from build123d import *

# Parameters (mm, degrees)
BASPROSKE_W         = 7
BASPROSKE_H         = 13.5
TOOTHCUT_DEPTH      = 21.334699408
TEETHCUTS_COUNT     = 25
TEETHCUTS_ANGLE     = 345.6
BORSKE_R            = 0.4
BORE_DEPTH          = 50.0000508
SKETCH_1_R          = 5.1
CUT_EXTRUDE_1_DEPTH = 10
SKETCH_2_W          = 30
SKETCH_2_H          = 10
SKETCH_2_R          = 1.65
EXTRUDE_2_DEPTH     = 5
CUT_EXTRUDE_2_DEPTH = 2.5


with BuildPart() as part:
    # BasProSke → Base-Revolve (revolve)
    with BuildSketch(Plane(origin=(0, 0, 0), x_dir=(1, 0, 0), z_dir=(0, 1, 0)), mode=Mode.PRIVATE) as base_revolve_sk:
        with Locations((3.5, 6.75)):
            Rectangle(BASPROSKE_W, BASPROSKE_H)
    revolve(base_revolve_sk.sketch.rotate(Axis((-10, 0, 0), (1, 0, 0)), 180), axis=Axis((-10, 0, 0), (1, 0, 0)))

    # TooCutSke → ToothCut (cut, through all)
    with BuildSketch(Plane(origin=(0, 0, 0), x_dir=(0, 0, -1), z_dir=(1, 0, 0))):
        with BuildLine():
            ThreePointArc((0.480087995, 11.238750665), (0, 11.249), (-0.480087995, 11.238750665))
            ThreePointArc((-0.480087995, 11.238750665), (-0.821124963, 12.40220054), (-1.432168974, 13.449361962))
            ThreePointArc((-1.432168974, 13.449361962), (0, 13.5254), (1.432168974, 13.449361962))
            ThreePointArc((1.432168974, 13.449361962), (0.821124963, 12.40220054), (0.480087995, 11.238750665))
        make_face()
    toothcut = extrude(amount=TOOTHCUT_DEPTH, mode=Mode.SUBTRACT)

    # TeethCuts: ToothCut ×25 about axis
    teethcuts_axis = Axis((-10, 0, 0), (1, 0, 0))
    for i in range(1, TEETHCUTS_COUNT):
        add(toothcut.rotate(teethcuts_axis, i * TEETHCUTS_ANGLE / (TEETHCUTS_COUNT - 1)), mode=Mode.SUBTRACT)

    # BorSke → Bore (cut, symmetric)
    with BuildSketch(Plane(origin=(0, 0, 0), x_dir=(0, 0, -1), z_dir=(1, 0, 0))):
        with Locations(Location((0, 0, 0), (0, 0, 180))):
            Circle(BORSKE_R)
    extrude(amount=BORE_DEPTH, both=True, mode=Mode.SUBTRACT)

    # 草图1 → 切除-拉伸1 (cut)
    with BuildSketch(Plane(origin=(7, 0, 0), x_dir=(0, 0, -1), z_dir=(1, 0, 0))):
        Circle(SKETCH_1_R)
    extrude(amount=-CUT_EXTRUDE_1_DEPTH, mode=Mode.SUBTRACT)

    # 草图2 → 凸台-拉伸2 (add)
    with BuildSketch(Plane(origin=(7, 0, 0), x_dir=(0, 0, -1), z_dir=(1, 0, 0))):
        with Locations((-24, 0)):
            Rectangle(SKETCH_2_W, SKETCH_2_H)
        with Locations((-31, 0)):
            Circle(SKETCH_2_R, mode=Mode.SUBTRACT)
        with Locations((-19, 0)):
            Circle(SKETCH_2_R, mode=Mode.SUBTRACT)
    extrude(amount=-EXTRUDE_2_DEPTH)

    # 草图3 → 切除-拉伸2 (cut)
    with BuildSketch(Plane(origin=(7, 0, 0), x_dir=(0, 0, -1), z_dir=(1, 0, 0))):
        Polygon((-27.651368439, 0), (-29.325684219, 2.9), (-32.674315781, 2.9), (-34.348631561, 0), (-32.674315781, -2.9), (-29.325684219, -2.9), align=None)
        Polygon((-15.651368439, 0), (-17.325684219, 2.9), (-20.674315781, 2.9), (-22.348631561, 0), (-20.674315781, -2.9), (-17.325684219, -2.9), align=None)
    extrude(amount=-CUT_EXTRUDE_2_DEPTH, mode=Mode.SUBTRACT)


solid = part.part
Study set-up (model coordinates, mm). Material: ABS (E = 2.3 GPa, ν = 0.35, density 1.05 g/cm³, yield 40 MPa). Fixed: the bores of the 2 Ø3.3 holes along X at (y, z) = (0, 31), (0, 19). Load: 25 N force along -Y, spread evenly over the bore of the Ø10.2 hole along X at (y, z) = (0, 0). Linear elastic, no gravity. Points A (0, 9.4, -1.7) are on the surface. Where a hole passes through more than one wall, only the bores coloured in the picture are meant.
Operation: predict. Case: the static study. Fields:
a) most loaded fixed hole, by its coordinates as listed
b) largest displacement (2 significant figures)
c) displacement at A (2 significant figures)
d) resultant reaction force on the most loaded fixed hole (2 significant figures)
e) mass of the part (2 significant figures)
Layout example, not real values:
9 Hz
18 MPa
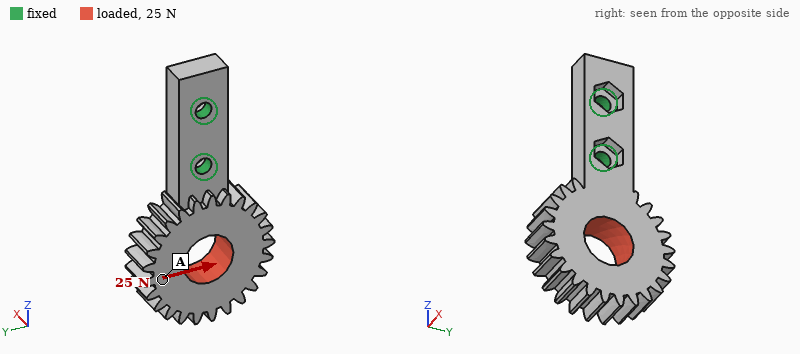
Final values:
(0, 19)
0.20 mm
0.14 mm
48 N
4.1 g
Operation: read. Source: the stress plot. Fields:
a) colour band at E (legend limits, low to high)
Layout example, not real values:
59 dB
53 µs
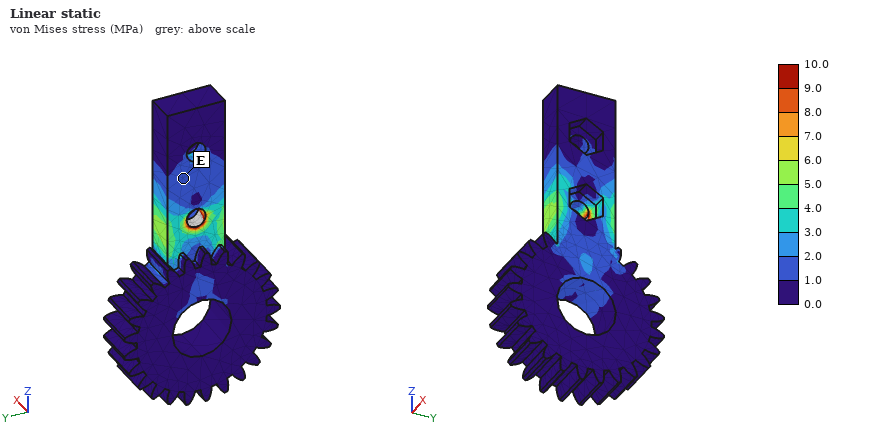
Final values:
1.0 to 2.0 MPa
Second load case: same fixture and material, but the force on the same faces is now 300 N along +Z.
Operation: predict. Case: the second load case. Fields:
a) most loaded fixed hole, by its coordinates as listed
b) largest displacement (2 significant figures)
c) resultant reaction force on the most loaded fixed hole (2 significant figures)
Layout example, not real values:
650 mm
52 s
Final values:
(0, 19)
0.20 mm
260 N
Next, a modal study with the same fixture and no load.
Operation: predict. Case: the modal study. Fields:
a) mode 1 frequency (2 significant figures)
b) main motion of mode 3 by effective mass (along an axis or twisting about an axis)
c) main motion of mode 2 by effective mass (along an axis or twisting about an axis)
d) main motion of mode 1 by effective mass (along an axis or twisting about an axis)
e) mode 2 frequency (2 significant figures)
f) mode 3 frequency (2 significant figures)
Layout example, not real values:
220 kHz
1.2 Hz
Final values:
720 Hz
twisting about Z
along Y
along X
1200 Hz
1700 Hz
